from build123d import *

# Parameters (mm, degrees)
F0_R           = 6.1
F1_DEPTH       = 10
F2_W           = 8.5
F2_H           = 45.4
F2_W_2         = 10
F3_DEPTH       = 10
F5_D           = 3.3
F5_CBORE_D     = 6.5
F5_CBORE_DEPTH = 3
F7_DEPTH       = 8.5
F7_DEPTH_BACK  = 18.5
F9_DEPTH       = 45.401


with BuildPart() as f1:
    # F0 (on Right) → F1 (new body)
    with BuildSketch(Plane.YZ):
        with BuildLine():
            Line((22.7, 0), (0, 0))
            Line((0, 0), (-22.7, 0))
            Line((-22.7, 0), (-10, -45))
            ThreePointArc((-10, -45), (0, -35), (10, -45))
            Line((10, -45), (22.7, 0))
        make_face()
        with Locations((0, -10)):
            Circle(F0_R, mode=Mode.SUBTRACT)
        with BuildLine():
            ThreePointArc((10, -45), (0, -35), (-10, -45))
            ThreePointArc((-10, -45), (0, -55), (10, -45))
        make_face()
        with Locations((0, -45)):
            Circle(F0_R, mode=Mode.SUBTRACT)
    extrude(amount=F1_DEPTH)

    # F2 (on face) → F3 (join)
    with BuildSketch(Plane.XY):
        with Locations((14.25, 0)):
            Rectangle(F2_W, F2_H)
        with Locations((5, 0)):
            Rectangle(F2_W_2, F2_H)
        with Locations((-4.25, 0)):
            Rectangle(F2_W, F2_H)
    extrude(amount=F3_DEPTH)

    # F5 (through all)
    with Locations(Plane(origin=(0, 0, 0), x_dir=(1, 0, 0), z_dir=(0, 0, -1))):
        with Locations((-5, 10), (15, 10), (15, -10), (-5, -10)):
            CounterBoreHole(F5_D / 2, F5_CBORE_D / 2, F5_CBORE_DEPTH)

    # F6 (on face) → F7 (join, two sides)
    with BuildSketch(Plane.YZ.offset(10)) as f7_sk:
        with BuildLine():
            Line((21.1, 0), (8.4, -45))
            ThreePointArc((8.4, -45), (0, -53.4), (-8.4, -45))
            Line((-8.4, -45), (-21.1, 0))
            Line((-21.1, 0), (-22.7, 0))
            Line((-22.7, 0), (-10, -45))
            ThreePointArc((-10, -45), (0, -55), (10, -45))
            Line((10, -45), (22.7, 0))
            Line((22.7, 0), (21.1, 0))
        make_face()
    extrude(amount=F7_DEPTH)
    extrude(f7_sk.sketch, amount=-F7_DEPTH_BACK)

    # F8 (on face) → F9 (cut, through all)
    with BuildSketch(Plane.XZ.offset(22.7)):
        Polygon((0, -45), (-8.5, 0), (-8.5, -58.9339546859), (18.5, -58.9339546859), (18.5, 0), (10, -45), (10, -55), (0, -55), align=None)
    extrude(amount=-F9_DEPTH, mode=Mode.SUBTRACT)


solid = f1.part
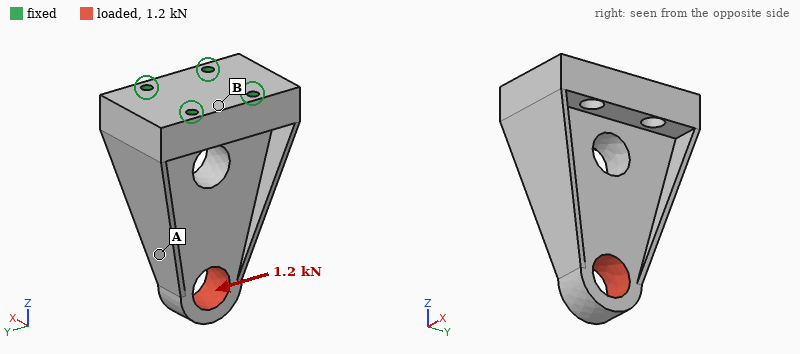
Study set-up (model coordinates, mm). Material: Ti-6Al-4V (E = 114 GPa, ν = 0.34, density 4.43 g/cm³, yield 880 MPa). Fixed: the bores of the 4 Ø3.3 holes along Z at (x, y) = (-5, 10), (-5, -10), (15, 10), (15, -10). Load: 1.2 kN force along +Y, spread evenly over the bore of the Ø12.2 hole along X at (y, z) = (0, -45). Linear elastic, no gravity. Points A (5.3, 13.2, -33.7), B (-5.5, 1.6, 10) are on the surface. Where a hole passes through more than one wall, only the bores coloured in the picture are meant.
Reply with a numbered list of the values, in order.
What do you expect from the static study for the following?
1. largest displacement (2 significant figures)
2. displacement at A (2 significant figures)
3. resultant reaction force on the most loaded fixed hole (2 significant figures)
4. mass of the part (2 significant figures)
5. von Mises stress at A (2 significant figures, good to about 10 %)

1. 34 µm
2. 19 µm
3. 1.3 kN
4. 120 g
5. 16 MPa
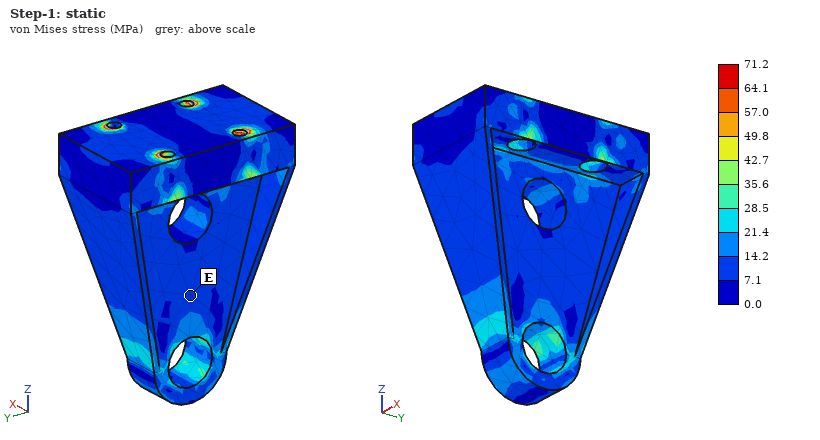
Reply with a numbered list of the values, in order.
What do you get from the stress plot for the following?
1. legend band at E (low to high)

1. 7.1 to 14.2 MPa
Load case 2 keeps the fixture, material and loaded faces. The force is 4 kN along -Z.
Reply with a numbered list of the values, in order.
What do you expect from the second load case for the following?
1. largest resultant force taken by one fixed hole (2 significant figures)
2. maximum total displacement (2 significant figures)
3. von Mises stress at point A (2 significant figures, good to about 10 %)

1. 1.0 kN
2. 13 µm
3. 21 MPa
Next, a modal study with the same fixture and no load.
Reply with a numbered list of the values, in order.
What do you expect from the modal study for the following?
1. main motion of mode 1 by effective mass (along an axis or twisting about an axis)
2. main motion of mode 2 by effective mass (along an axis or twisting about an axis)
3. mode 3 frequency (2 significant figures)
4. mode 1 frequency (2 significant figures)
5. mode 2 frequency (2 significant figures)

1. along X
2. along Y
3. 12 kHz
4. 4100 Hz
5. 7000 Hz
